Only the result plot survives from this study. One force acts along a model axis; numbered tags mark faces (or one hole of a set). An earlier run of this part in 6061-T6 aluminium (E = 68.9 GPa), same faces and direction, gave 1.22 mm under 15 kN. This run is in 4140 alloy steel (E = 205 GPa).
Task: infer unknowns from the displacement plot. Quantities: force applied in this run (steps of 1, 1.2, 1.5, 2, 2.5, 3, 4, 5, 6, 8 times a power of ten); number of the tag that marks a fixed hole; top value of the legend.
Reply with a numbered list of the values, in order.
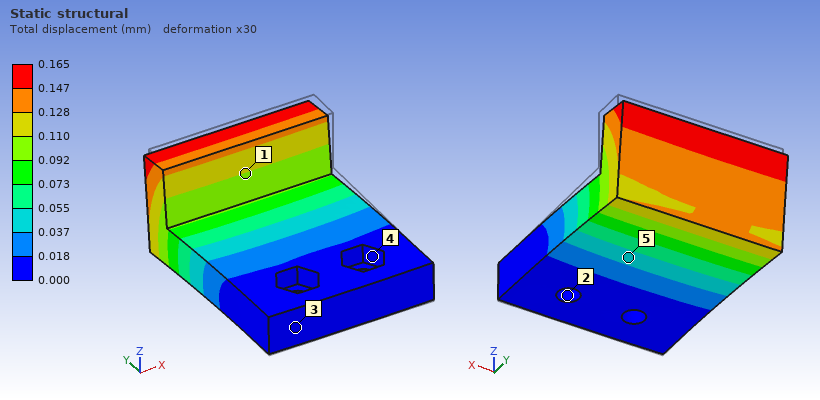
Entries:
1. 6 kN
2. 2
3. 0.165 mm
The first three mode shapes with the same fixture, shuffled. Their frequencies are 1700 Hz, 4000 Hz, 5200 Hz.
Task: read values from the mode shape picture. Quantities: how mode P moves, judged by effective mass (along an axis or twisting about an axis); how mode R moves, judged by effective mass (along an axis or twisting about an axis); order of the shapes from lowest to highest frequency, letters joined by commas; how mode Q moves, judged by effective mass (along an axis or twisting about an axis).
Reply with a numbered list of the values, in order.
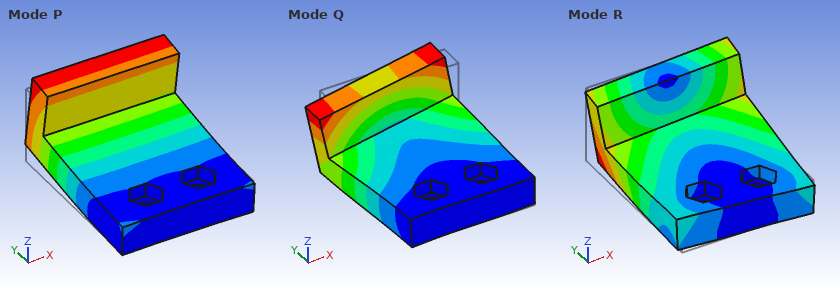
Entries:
1. along Z
2. along X
3. P, Q, R
4. along X
